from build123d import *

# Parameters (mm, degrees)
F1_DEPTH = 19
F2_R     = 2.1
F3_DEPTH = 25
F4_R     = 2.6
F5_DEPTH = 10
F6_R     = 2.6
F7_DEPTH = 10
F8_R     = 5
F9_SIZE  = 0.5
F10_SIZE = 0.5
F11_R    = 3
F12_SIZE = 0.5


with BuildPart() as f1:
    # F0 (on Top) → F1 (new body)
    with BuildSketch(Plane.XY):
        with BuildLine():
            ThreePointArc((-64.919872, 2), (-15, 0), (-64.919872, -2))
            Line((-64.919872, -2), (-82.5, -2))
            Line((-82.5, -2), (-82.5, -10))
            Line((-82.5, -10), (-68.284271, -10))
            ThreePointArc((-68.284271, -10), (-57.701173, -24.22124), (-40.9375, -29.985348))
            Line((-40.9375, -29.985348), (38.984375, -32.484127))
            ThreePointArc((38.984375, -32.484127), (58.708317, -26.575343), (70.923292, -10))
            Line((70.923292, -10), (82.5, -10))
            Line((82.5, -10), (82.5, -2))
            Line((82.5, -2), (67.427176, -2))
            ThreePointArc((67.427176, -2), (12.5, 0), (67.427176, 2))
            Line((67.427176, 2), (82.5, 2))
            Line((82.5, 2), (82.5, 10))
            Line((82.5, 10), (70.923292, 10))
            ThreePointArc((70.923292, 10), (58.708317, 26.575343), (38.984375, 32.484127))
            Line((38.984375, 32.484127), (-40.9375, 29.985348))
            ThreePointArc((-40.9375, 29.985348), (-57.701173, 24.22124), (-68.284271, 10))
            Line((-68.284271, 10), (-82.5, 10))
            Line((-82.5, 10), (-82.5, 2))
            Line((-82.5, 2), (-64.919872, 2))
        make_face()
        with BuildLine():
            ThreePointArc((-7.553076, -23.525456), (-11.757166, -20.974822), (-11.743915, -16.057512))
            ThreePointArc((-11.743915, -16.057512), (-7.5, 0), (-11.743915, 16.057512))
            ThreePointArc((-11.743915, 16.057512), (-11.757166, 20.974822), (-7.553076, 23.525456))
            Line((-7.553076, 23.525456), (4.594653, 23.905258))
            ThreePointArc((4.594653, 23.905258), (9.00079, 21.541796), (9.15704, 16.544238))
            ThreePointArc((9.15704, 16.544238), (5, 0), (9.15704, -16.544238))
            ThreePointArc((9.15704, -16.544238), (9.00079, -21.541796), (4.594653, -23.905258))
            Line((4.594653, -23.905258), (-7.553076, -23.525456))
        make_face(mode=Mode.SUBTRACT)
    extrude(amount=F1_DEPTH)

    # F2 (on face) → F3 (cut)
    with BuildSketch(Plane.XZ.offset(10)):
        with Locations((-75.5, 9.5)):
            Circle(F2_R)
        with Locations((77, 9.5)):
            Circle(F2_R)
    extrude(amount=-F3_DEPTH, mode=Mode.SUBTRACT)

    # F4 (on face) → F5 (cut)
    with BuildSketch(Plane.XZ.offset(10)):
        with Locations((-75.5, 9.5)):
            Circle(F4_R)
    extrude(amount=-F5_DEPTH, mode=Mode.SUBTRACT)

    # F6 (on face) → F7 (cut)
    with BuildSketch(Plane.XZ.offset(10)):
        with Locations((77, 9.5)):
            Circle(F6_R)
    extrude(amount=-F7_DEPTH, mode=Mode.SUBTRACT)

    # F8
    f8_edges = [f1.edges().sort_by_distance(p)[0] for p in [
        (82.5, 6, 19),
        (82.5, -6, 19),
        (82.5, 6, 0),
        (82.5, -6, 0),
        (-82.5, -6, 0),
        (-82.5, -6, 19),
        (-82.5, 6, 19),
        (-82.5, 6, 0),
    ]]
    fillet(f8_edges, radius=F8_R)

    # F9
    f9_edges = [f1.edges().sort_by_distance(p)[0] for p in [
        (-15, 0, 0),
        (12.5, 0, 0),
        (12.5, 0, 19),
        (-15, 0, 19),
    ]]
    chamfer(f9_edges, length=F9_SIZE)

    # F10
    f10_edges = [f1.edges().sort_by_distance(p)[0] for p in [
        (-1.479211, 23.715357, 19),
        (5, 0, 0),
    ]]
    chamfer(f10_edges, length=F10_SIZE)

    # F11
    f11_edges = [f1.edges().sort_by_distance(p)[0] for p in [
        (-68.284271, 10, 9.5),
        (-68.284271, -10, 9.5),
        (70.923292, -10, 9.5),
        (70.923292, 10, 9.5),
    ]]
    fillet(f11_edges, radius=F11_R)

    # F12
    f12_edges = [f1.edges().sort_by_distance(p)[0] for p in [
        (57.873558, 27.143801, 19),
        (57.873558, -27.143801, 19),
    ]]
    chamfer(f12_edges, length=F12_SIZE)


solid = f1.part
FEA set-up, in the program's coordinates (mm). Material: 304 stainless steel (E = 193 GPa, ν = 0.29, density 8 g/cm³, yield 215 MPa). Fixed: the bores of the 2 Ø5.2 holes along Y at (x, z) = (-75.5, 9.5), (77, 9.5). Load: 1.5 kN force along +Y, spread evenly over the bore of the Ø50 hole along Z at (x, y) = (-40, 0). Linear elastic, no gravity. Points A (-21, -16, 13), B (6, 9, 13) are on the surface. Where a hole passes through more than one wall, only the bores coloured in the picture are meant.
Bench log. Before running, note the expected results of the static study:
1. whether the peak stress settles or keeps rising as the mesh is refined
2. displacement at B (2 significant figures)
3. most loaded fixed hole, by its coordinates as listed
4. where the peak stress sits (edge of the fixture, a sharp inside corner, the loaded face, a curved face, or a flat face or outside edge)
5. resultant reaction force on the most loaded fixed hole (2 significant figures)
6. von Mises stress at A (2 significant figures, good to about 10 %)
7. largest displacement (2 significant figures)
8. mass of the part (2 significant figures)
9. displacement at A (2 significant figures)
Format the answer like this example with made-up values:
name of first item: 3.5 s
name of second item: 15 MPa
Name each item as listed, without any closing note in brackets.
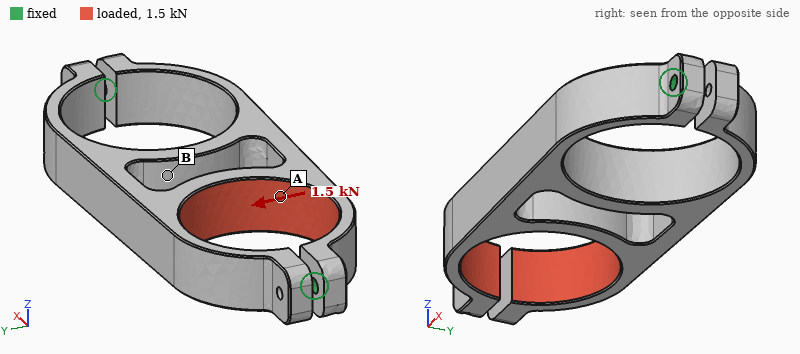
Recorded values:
whether the peak stress settles or keeps rising as the mesh is refined: keeps rising
displacement at B: 0.11 mm
most loaded fixed hole, by its coordinates as listed: (-75.5, 9.5)
where the peak stress sits: edge of the fixture
resultant reaction force on the most loaded fixed hole: 1.6 kN
von Mises stress at A: 40 MPa
largest displacement: 0.43 mm
mass of the part: 490 g
displacement at A: 0.098 mm
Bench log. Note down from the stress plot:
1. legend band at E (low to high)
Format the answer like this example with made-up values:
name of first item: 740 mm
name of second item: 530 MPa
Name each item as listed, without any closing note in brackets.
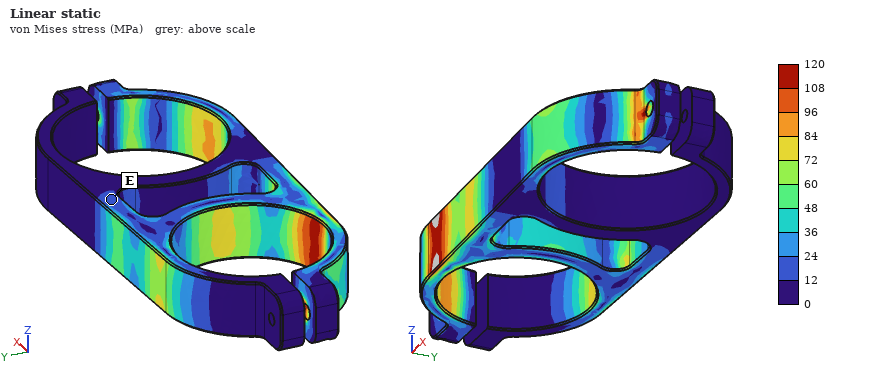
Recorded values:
legend band at E: 12 to 24 MPa
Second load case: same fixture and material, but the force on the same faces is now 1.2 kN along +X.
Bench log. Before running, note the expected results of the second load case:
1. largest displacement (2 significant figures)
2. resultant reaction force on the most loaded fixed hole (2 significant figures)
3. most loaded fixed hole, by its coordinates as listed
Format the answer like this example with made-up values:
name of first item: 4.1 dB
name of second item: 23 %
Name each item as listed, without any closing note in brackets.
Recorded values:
largest displacement: 0.21 mm
resultant reaction force on the most loaded fixed hole: 860 N
most loaded fixed hole, by its coordinates as listed: (-75.5, 9.5)
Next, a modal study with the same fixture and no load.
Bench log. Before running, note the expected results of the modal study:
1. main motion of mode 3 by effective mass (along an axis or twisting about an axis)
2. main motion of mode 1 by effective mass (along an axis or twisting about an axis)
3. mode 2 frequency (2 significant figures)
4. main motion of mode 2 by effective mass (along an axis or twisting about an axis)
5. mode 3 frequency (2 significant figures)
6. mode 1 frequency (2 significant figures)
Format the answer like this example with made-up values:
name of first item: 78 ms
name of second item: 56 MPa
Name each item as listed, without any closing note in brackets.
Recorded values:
main motion of mode 3 by effective mass: twisting about Y
main motion of mode 1 by effective mass: along Z
mode 2 frequency: 580 Hz
main motion of mode 2 by effective mass: along X
mode 3 frequency: 740 Hz
mode 1 frequency: 380 Hz
